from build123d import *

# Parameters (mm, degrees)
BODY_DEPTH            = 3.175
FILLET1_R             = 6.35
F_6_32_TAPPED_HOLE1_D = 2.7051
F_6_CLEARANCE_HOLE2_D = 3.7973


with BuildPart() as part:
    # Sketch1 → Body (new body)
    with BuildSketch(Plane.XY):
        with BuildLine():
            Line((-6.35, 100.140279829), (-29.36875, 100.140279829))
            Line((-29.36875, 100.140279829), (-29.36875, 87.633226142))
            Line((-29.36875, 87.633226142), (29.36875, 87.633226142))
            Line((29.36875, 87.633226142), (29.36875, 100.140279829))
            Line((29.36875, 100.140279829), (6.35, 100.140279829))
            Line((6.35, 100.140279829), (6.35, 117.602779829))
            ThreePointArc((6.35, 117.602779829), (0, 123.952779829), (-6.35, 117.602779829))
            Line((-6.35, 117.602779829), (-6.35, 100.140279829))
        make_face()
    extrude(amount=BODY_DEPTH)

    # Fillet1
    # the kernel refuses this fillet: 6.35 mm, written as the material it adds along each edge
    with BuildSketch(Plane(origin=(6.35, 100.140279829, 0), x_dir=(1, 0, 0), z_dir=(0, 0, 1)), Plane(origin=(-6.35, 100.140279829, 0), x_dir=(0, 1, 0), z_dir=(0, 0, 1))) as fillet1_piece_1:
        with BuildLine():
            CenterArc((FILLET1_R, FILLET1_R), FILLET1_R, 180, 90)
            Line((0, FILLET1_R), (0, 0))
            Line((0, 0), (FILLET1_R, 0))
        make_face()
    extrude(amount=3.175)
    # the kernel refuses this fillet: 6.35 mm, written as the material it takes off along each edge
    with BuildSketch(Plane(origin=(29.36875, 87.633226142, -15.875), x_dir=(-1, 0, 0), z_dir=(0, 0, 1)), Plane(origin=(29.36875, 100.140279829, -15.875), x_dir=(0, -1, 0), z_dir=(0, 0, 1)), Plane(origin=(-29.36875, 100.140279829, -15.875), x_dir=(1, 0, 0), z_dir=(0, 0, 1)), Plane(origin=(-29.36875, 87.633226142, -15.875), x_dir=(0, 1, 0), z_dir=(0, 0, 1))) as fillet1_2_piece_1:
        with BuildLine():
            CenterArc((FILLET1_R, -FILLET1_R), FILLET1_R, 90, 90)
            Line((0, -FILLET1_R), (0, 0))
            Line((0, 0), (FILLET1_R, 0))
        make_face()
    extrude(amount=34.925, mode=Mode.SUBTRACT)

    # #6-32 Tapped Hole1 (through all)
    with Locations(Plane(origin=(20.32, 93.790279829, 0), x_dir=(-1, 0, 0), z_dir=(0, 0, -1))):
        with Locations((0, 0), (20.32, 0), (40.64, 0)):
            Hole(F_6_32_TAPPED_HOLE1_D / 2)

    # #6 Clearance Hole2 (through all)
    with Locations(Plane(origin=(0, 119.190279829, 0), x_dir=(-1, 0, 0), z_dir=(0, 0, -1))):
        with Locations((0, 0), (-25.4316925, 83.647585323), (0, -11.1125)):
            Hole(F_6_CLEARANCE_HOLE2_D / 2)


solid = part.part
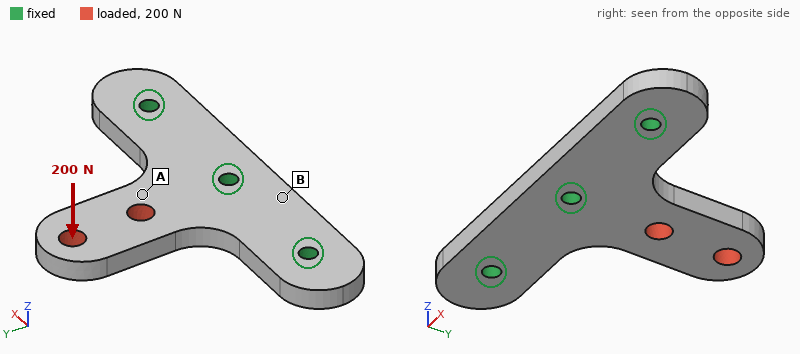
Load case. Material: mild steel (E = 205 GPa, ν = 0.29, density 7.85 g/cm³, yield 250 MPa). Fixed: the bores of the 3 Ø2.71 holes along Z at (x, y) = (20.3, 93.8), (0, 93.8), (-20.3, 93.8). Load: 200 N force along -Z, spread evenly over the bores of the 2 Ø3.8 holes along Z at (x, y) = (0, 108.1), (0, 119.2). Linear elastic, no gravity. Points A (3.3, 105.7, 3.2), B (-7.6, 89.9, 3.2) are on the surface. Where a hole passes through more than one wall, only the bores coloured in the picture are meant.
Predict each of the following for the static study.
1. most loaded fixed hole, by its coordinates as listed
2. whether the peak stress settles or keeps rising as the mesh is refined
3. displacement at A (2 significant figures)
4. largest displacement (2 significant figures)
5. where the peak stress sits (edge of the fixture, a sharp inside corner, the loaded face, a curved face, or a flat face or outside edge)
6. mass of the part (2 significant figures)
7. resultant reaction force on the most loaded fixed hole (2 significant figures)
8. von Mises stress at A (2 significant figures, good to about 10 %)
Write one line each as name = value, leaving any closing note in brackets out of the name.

most loaded fixed hole, by its coordinates as listed = (0, 93.8)
whether the peak stress settles or keeps rising as the mesh is refined = keeps rising
displacement at A = 0.023 mm
largest displacement = 0.11 mm
where the peak stress sits = edge of the fixture
mass of the part = 24 g
resultant reaction force on the most loaded fixed hole = 210 N
von Mises stress at A = 87 MPa
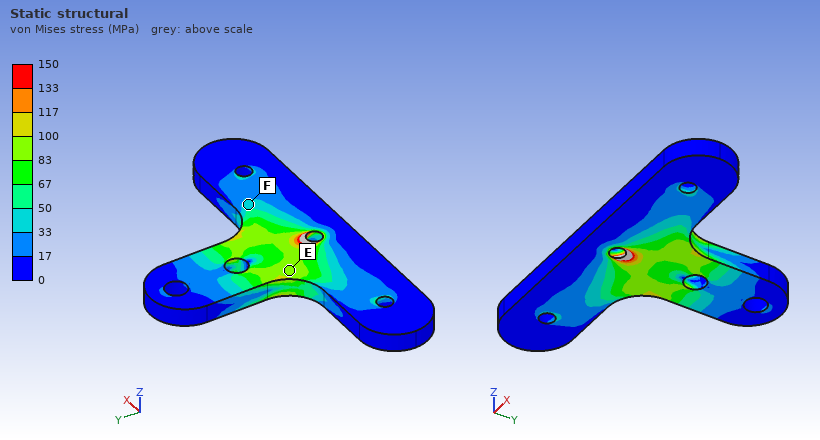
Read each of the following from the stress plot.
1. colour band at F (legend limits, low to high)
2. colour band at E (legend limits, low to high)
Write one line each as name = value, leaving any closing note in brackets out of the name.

colour band at F = 33 to 50 MPa
colour band at E = 83 to 100 MPa
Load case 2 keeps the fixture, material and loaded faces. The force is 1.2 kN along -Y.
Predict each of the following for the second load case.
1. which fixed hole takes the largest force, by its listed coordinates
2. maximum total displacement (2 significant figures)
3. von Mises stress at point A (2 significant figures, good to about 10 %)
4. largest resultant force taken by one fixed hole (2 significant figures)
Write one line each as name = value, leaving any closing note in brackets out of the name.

which fixed hole takes the largest force, by its listed coordinates = (0, 93.8)
maximum total displacement = 3.7 µm
von Mises stress at point A = 33 MPa
largest resultant force taken by one fixed hole = 980 N
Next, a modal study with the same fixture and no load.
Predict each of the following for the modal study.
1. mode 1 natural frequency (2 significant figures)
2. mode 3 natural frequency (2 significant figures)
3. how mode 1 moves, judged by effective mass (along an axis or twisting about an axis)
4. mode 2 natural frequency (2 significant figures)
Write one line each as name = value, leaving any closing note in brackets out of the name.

mode 1 natural frequency = 3700 Hz
mode 3 natural frequency = 15 kHz
how mode 1 moves, judged by effective mass = along Z
mode 2 natural frequency = 15 kHz
